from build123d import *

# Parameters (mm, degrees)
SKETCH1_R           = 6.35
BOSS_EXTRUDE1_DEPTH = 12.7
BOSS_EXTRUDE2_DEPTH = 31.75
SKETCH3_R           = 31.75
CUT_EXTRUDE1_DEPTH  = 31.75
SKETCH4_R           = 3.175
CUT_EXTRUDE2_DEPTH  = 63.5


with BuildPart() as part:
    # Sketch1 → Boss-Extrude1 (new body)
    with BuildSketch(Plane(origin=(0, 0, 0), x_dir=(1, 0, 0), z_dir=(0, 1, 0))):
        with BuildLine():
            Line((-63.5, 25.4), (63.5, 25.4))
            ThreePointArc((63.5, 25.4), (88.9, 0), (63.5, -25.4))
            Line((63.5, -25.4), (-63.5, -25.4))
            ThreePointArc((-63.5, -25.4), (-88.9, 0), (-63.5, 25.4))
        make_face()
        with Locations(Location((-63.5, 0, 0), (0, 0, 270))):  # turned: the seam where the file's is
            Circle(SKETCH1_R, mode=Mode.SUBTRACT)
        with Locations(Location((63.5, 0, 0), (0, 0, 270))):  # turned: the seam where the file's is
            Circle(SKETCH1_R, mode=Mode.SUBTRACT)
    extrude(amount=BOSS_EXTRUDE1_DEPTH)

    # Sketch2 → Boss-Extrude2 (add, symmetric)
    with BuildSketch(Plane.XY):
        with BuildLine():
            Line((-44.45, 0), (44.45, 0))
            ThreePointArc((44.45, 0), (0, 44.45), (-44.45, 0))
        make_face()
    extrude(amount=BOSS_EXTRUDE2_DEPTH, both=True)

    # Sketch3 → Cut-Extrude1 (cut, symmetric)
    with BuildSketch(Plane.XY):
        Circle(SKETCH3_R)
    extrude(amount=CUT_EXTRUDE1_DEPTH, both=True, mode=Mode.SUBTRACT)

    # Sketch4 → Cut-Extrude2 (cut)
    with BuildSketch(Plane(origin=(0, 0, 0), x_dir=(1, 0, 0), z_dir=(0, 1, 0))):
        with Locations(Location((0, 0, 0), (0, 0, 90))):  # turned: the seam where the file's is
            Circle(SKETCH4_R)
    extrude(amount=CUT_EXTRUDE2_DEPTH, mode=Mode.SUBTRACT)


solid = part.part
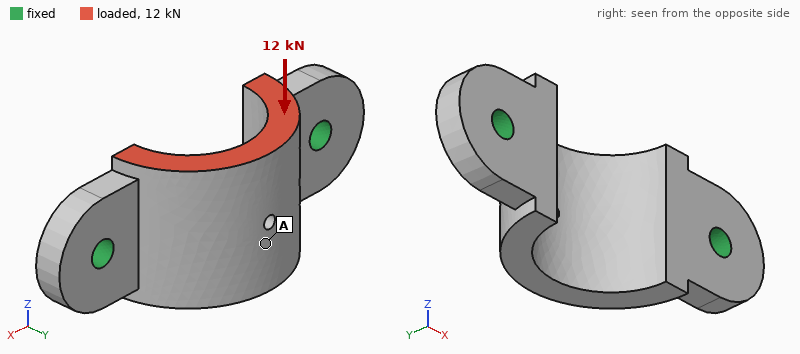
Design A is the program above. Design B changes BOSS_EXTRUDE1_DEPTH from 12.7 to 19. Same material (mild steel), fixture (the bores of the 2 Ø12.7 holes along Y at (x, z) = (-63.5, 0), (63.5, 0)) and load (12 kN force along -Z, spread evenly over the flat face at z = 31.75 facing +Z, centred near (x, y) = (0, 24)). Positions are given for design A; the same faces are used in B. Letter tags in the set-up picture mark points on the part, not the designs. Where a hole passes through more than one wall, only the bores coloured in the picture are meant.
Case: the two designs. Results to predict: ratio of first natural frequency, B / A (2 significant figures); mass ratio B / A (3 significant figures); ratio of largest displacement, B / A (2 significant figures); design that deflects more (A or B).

1.5
1.18
0.49
A
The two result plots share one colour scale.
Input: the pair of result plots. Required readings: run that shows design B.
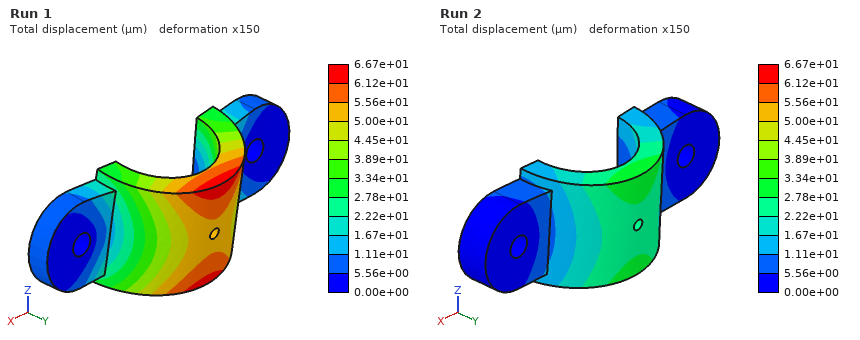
Run 2
